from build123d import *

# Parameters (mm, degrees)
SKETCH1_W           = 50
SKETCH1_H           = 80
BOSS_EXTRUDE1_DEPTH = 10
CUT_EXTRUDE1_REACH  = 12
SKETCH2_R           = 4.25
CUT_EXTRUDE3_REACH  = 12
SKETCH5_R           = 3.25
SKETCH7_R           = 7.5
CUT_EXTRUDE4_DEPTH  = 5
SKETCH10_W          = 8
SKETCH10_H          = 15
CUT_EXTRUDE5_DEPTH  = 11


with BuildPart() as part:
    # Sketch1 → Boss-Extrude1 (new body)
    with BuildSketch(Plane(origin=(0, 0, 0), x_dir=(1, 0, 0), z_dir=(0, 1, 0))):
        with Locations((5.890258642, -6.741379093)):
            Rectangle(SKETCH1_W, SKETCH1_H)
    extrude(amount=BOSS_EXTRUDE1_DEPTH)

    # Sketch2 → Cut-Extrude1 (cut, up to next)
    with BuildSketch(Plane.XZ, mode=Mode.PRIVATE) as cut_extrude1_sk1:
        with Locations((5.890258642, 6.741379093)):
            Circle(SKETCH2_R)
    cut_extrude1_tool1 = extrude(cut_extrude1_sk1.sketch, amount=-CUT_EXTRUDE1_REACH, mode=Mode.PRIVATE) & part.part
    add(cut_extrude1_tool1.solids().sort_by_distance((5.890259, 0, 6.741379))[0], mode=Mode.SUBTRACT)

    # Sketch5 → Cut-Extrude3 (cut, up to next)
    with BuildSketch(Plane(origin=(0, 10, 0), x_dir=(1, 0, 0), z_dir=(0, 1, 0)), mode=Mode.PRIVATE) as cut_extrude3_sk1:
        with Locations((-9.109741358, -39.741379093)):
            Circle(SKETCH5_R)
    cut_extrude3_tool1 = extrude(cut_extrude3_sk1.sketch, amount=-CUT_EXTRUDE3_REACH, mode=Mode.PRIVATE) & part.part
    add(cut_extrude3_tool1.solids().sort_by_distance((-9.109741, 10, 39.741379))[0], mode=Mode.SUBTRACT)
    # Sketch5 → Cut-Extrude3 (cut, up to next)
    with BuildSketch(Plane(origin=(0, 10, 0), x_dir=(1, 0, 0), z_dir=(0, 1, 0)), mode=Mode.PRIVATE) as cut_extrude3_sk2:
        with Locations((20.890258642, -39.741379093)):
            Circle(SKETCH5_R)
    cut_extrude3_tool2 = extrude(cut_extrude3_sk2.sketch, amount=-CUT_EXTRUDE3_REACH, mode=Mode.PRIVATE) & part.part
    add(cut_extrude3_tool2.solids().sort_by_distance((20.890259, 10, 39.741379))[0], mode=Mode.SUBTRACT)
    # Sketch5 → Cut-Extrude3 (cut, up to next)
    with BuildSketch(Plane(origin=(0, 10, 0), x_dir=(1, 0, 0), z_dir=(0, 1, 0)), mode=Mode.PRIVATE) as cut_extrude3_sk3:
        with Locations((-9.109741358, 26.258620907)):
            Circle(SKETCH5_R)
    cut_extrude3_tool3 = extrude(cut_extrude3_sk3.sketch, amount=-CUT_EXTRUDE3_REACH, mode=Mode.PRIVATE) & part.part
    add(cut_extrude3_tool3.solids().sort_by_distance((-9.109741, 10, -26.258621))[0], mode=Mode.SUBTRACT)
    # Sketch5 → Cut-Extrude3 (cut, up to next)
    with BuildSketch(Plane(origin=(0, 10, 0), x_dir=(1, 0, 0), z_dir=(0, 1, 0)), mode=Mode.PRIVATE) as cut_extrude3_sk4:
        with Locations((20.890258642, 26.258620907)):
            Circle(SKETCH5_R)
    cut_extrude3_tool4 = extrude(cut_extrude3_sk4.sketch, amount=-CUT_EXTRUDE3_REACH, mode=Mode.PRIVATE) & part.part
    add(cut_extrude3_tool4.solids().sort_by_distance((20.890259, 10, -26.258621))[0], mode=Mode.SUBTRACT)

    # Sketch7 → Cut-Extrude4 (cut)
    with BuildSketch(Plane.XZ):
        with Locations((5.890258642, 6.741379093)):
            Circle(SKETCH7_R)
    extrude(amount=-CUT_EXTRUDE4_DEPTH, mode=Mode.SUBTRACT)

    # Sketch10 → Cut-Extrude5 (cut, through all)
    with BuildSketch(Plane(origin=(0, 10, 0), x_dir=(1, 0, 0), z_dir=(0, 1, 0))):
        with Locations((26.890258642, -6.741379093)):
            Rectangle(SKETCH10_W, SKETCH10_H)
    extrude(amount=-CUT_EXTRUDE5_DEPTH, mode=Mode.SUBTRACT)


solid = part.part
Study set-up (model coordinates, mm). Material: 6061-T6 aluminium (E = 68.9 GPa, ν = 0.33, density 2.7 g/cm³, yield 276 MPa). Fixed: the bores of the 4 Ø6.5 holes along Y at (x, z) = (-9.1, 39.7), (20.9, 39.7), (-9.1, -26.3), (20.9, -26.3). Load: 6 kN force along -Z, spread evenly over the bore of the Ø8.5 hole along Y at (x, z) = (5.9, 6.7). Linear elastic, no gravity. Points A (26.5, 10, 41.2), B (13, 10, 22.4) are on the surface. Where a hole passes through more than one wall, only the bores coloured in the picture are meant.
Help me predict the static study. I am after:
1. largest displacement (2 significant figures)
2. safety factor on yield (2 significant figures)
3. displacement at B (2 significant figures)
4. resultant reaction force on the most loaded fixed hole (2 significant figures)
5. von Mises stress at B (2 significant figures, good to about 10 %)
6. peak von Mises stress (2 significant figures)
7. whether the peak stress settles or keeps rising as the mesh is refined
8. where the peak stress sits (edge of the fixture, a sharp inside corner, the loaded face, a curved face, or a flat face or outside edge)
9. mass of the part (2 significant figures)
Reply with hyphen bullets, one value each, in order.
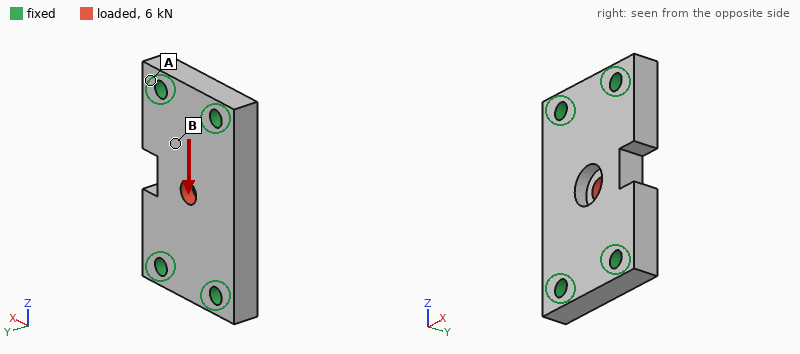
- 8.7 µm
- 3.4
- 2.7 µm
- 1.6 kN
- 16 MPa
- 81 MPa
- settles
- the loaded face
- 98 g
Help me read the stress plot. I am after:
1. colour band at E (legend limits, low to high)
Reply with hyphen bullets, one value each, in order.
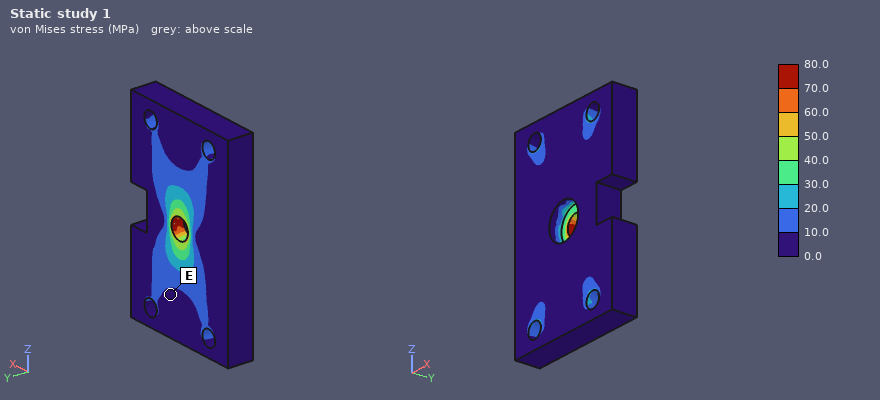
- 0.0 to 10.0 MPa
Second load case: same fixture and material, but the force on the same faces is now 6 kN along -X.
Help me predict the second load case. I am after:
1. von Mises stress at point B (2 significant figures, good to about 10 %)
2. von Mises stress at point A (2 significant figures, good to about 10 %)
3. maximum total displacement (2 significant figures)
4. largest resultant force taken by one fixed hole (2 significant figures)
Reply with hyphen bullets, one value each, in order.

- 19 MPa
- 7.5 MPa
- 16 µm
- 2.2 kN
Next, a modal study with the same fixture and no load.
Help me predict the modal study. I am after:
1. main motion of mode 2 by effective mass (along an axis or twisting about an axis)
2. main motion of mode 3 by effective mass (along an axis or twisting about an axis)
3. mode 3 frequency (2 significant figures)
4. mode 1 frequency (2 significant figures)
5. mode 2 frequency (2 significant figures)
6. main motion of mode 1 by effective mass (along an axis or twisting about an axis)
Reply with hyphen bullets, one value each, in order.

- twisting about Z
- along X
- 21 kHz
- 11 kHz
- 14 kHz
- along Y
